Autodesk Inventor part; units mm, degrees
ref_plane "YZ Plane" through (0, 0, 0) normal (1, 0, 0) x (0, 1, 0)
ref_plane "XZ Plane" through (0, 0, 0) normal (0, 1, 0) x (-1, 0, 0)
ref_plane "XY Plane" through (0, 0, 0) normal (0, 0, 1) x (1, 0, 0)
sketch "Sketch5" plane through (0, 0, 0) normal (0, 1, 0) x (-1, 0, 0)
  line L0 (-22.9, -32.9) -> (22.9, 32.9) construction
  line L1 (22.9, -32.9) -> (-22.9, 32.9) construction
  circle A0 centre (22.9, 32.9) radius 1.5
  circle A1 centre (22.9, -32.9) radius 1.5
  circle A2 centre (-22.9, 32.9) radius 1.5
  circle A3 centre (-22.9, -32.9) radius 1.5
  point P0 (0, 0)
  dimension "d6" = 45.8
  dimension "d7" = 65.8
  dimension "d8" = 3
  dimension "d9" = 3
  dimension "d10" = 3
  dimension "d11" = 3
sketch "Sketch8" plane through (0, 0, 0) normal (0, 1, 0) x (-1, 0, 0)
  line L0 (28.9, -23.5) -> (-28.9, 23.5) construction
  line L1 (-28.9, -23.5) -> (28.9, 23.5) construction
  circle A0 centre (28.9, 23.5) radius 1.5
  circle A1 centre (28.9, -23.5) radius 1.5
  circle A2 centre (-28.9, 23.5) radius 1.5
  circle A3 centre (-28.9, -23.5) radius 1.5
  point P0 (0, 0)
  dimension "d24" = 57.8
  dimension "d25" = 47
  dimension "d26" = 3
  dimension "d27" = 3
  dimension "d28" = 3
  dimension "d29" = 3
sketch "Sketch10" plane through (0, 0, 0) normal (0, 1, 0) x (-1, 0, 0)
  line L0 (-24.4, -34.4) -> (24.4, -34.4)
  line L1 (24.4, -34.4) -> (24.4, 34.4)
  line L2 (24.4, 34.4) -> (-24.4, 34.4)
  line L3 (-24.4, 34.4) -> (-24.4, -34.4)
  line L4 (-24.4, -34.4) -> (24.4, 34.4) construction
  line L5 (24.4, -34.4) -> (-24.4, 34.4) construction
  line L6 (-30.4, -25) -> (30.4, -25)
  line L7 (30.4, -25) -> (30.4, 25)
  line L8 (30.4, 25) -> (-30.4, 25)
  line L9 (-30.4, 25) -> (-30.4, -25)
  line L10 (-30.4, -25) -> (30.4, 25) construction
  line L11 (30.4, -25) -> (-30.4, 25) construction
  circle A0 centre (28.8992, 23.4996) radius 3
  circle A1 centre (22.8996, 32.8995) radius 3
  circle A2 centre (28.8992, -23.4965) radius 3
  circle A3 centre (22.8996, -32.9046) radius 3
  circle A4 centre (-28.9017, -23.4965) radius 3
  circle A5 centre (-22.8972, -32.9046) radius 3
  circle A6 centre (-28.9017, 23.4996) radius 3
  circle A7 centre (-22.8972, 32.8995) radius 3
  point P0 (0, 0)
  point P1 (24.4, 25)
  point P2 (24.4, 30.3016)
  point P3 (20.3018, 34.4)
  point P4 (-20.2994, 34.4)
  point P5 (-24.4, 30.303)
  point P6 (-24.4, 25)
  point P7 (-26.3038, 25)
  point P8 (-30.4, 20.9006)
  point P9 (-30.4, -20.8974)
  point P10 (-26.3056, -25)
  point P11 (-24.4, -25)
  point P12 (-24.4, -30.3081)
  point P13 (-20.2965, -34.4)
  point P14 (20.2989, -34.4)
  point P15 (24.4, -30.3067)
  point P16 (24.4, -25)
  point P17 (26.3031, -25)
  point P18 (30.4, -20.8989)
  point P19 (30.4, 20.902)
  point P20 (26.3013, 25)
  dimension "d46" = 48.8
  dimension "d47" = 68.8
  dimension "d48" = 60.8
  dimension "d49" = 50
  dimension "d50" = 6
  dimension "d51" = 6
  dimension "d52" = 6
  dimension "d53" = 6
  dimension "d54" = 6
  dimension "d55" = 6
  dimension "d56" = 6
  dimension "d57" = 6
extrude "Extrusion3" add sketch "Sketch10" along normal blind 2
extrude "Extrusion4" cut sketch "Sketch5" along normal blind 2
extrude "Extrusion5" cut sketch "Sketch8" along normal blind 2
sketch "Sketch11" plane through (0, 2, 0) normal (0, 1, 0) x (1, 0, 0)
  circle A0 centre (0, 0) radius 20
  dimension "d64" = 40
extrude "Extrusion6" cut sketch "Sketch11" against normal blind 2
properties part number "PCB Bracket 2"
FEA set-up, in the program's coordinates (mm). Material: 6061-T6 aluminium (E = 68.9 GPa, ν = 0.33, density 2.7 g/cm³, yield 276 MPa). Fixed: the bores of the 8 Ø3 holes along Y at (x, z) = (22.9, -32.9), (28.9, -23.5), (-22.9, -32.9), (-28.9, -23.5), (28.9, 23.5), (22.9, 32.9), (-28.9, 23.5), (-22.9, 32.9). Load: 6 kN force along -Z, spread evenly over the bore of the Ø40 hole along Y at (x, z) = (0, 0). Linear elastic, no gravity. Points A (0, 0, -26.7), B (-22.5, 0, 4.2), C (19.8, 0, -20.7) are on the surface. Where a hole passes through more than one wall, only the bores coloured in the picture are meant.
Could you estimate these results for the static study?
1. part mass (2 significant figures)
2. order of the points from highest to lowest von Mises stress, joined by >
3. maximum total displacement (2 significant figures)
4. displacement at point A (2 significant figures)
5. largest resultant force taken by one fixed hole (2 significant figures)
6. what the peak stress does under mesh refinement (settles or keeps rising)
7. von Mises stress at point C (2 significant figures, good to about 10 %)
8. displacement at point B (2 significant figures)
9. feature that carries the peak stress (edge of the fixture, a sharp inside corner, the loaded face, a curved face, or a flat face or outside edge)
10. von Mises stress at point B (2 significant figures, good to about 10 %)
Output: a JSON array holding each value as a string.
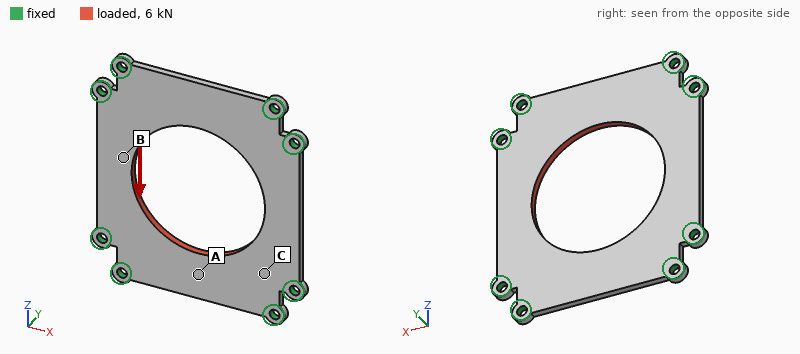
["15 g", "B > C > A", "29 µm", "28 µm", "1.1 kN", "keeps rising", "30 MPa", "12 µm", "edge of the fixture", "42 MPa"]
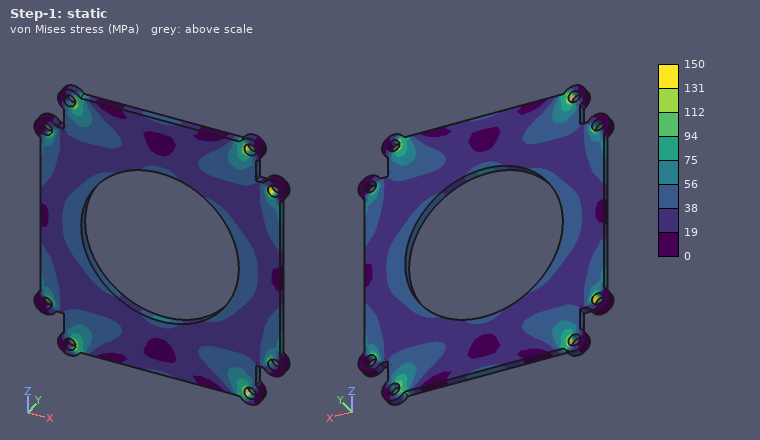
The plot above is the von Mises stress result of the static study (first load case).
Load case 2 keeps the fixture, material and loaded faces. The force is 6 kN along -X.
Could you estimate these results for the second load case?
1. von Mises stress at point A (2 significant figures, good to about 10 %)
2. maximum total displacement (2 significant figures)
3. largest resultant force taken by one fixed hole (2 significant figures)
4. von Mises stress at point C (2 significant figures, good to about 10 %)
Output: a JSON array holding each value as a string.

["41 MPa", "40 µm", "1.2 kN", "42 MPa"]
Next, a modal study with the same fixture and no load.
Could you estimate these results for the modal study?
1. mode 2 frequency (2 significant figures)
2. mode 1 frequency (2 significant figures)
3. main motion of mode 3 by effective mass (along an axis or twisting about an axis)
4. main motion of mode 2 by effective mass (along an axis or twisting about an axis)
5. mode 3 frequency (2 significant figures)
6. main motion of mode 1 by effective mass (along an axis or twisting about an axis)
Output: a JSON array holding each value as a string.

["4500 Hz", "3800 Hz", "twisting about Z", "twisting about X", "4800 Hz", "along Y"]
